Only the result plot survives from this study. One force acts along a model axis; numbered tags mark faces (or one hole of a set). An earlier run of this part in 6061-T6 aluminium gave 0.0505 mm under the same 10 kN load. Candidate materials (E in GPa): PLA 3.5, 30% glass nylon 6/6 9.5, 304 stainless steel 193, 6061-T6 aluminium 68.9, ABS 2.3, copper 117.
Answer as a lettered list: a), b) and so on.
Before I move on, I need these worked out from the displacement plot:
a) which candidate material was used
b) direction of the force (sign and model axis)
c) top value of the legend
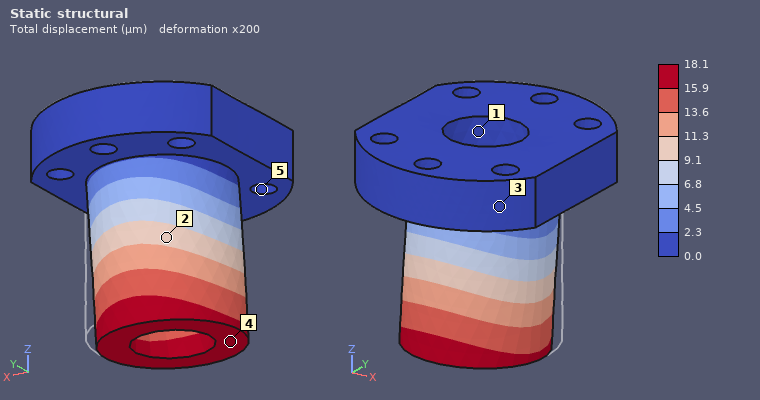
a) 304 stainless steel
b) -Y
c) 18.1 µm
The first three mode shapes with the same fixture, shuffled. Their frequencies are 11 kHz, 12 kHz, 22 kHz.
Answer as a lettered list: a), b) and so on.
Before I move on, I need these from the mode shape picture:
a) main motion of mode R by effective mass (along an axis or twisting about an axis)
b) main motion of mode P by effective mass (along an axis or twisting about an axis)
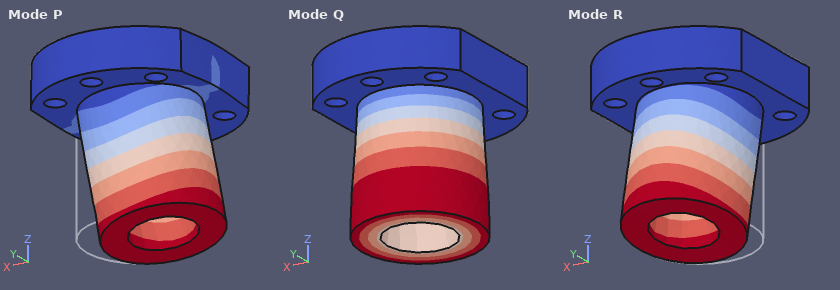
a) along Y
b) along X
